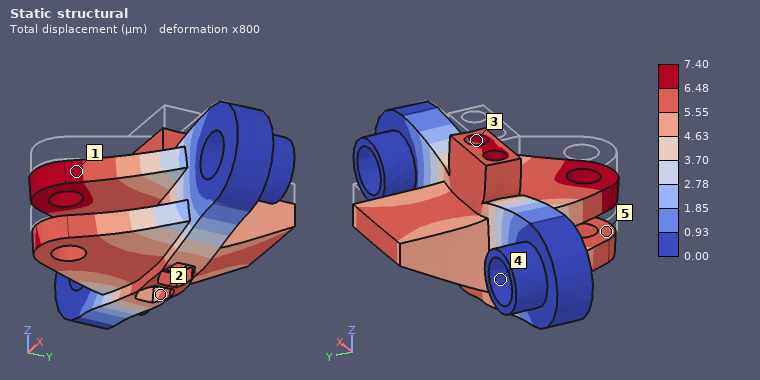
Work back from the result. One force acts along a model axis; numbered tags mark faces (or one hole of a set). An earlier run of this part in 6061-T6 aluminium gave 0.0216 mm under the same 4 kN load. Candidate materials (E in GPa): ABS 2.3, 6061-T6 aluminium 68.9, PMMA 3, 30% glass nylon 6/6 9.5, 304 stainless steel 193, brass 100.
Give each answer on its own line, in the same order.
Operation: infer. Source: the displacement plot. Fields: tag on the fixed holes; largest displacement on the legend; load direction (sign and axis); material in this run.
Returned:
4
7.40 µm
-Z
304 stainless steel
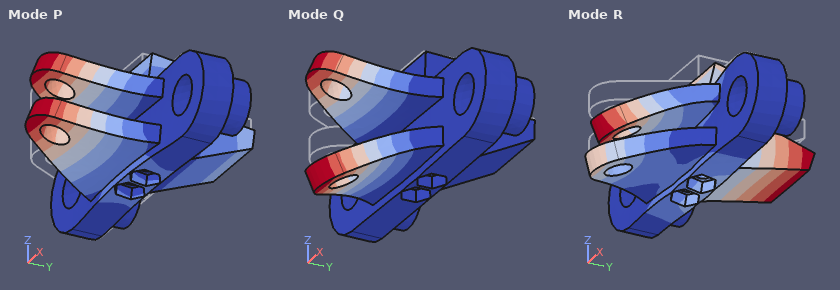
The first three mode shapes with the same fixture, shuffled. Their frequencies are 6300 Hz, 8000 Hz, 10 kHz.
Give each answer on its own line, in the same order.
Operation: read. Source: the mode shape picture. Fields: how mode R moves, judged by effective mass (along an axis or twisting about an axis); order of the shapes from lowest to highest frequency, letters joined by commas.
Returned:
along Z
P, Q, R
